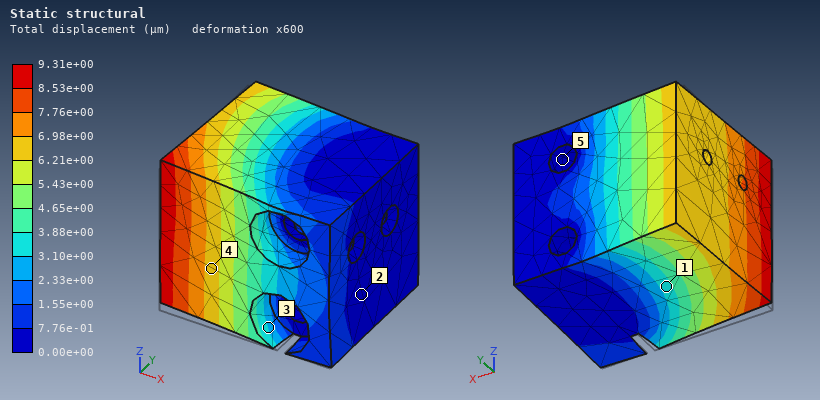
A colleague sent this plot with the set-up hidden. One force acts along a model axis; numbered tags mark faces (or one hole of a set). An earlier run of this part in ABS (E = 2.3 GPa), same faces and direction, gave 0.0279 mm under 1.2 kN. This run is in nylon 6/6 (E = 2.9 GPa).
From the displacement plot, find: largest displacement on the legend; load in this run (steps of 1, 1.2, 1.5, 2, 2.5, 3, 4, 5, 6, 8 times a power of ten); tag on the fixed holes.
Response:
9.31e+00 µm
500 N
5
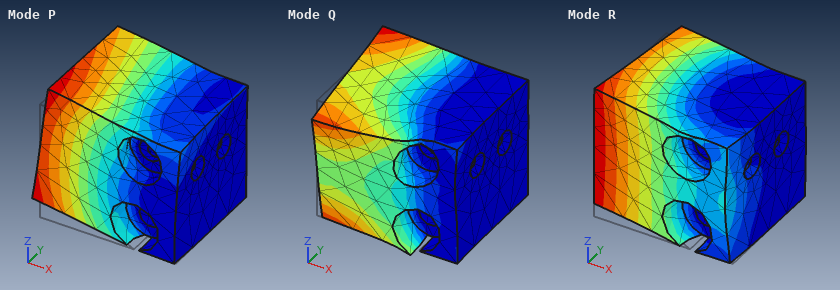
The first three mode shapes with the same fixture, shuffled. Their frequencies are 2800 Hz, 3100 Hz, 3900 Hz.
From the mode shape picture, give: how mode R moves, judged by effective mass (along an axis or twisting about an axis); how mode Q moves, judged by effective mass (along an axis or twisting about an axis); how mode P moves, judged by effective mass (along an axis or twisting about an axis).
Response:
along Y
twisting about X
along Z
